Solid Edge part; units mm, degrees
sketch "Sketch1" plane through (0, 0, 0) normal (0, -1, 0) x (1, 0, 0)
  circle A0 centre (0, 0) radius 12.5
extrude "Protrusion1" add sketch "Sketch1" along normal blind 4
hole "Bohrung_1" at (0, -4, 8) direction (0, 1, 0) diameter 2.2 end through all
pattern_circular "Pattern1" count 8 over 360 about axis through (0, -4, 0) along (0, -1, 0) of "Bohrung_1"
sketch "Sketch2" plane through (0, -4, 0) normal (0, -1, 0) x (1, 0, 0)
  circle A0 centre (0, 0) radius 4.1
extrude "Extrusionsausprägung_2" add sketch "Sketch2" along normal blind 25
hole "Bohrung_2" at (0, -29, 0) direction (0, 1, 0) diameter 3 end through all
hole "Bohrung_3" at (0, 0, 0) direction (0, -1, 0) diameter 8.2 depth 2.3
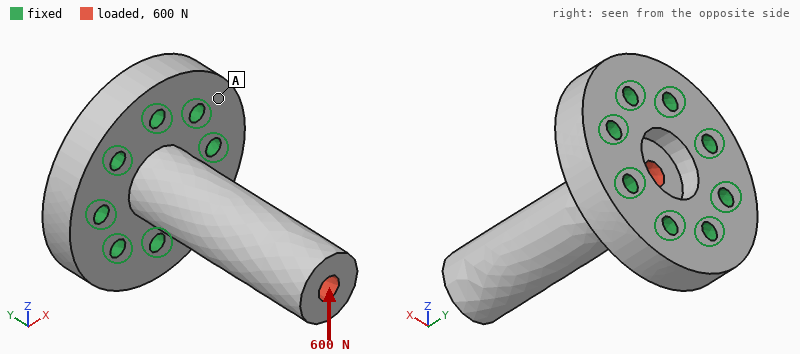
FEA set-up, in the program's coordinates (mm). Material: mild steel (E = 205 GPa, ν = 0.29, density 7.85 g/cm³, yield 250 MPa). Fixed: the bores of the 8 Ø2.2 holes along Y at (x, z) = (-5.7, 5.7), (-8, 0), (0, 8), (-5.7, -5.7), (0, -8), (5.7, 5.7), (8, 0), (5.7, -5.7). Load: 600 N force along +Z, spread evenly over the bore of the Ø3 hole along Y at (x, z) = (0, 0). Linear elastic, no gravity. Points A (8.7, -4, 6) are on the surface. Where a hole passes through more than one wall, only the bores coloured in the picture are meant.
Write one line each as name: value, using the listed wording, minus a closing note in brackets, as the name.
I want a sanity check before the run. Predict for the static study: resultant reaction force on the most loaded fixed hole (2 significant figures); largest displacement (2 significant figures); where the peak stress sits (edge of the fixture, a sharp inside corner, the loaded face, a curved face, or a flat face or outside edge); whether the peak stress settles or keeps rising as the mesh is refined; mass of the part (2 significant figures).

resultant reaction force on the most loaded fixed hole: 390 N
largest displacement: 43 µm
where the peak stress sits: a sharp inside corner
whether the peak stress settles or keeps rising as the mesh is refined: keeps rising
mass of the part: 22 g
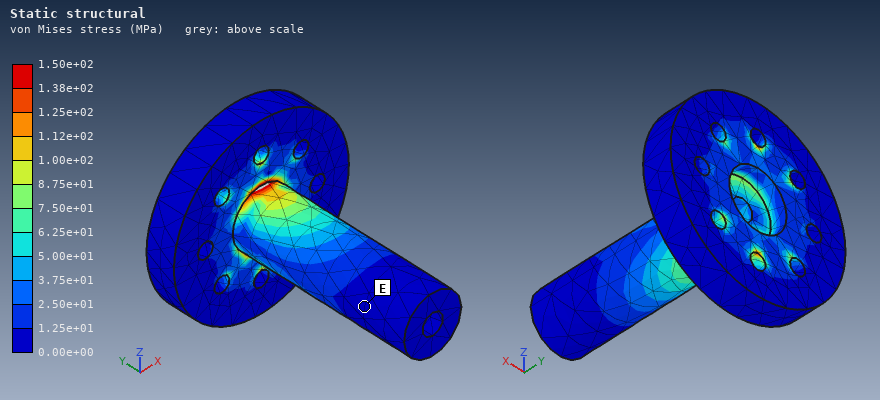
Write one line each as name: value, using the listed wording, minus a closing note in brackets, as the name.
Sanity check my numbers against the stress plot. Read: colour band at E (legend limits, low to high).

colour band at E: 0.00e+00 to 1.25e+01 MPa
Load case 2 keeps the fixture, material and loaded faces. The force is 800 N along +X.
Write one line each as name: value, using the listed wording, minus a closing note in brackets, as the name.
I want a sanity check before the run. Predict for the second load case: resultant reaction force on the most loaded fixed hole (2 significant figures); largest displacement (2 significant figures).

resultant reaction force on the most loaded fixed hole: 520 N
largest displacement: 57 µm
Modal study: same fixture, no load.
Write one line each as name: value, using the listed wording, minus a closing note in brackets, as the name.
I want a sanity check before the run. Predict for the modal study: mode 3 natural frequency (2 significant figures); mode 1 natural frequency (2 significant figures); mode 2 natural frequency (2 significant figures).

mode 3 natural frequency: 30 kHz
mode 1 natural frequency: 7500 Hz
mode 2 natural frequency: 7500 Hz
